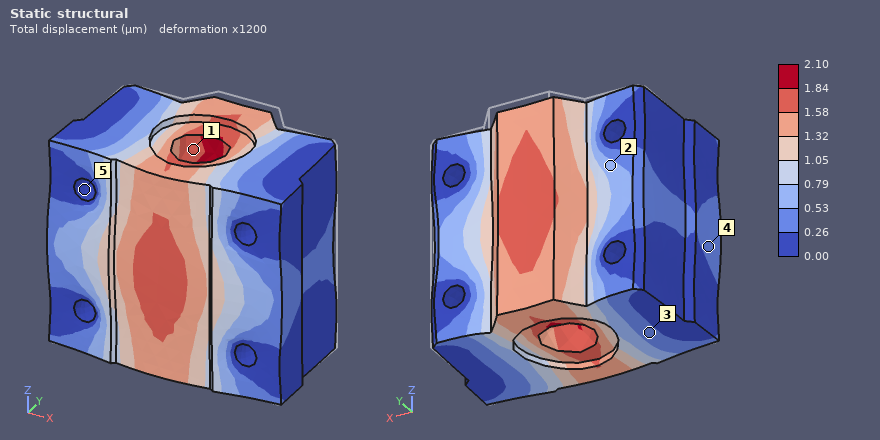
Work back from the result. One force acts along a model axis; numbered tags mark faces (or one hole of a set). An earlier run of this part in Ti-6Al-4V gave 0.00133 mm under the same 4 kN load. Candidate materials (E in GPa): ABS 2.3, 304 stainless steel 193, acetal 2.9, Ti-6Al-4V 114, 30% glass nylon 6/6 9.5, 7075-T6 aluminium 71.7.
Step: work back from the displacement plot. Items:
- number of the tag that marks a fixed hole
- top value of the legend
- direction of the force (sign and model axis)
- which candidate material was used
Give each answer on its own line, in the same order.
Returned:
5
2.10 µm
-Y
7075-T6 aluminium
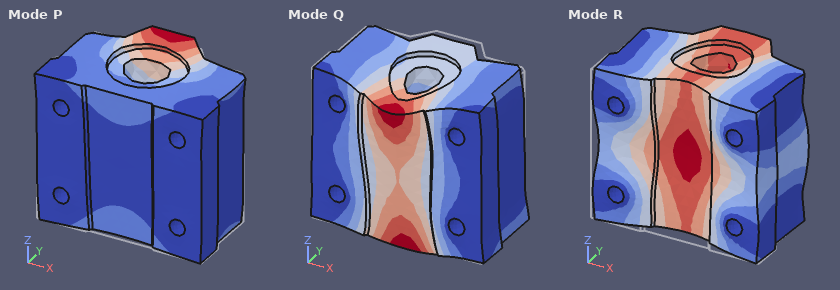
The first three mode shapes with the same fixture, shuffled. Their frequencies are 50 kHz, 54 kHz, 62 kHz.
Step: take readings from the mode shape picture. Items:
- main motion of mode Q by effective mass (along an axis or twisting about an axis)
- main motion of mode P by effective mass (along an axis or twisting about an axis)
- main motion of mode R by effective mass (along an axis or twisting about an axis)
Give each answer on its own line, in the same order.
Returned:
along Z
along Z
along Y
